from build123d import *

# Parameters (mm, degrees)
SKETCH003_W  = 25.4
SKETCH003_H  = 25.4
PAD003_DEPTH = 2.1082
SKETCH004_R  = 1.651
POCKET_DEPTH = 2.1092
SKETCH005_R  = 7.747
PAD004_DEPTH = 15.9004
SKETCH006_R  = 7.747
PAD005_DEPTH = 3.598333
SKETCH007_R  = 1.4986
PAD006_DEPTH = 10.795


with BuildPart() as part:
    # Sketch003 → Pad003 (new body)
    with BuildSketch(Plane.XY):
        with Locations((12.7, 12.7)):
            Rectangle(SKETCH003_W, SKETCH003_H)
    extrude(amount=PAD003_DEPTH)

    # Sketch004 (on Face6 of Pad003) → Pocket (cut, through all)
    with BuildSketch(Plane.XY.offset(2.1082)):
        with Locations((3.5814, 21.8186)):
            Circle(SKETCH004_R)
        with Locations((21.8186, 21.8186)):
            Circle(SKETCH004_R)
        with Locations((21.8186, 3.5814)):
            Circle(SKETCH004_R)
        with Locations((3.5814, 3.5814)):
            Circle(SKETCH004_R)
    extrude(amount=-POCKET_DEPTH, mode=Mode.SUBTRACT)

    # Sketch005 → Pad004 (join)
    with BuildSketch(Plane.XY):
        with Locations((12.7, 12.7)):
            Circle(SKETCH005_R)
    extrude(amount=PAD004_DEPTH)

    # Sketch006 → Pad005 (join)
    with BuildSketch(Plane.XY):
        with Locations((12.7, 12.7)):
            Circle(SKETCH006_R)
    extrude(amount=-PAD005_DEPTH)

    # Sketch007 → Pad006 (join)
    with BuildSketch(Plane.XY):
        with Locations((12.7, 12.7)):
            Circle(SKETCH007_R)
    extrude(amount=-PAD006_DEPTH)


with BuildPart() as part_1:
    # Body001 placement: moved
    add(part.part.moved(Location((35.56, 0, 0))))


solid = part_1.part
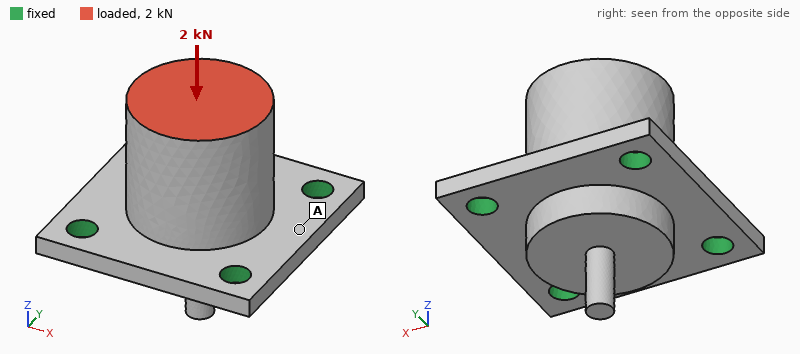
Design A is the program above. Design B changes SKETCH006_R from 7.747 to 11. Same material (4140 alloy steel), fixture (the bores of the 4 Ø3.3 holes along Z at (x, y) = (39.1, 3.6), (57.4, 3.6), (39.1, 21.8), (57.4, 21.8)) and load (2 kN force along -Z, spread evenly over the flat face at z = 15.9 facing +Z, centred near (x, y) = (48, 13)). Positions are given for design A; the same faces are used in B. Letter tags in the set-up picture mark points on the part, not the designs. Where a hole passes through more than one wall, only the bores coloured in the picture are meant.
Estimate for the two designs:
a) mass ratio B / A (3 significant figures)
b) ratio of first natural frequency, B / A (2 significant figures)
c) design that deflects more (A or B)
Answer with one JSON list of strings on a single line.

["1.15", "1.4", "A"]
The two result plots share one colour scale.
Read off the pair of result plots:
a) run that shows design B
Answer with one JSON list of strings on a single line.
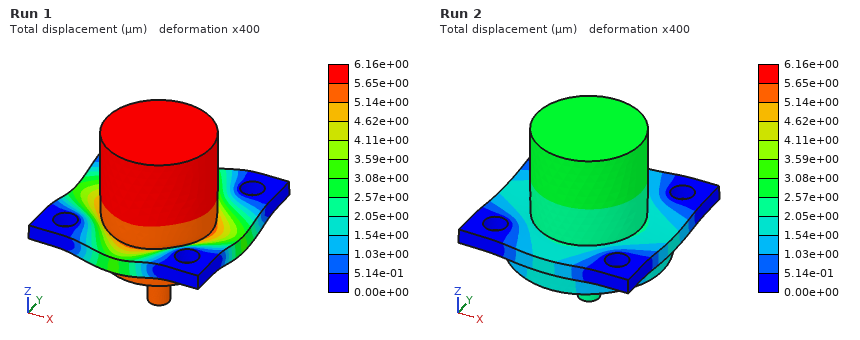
["Run 2"]
